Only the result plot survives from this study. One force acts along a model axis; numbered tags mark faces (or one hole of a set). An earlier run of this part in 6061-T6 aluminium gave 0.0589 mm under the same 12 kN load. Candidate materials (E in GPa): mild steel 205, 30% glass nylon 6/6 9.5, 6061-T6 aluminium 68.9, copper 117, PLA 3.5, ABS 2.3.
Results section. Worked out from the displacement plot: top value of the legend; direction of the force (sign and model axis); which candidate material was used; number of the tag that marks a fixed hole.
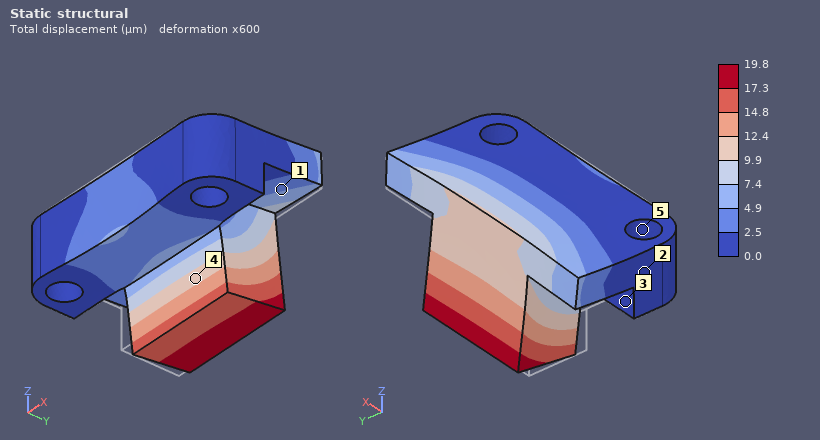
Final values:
19.8 µm
+Y
mild steel
5
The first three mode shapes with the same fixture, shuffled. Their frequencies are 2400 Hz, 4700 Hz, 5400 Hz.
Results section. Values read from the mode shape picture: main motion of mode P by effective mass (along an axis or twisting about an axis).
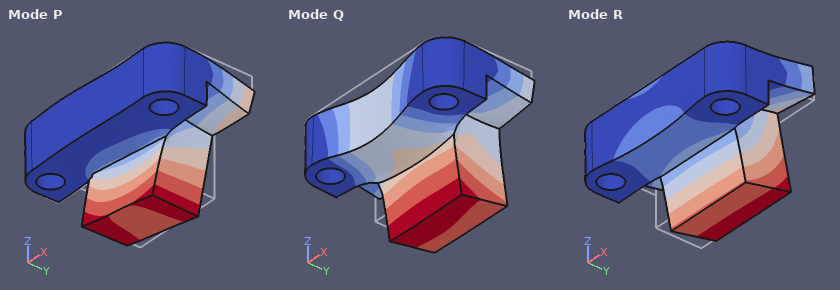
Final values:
along X
